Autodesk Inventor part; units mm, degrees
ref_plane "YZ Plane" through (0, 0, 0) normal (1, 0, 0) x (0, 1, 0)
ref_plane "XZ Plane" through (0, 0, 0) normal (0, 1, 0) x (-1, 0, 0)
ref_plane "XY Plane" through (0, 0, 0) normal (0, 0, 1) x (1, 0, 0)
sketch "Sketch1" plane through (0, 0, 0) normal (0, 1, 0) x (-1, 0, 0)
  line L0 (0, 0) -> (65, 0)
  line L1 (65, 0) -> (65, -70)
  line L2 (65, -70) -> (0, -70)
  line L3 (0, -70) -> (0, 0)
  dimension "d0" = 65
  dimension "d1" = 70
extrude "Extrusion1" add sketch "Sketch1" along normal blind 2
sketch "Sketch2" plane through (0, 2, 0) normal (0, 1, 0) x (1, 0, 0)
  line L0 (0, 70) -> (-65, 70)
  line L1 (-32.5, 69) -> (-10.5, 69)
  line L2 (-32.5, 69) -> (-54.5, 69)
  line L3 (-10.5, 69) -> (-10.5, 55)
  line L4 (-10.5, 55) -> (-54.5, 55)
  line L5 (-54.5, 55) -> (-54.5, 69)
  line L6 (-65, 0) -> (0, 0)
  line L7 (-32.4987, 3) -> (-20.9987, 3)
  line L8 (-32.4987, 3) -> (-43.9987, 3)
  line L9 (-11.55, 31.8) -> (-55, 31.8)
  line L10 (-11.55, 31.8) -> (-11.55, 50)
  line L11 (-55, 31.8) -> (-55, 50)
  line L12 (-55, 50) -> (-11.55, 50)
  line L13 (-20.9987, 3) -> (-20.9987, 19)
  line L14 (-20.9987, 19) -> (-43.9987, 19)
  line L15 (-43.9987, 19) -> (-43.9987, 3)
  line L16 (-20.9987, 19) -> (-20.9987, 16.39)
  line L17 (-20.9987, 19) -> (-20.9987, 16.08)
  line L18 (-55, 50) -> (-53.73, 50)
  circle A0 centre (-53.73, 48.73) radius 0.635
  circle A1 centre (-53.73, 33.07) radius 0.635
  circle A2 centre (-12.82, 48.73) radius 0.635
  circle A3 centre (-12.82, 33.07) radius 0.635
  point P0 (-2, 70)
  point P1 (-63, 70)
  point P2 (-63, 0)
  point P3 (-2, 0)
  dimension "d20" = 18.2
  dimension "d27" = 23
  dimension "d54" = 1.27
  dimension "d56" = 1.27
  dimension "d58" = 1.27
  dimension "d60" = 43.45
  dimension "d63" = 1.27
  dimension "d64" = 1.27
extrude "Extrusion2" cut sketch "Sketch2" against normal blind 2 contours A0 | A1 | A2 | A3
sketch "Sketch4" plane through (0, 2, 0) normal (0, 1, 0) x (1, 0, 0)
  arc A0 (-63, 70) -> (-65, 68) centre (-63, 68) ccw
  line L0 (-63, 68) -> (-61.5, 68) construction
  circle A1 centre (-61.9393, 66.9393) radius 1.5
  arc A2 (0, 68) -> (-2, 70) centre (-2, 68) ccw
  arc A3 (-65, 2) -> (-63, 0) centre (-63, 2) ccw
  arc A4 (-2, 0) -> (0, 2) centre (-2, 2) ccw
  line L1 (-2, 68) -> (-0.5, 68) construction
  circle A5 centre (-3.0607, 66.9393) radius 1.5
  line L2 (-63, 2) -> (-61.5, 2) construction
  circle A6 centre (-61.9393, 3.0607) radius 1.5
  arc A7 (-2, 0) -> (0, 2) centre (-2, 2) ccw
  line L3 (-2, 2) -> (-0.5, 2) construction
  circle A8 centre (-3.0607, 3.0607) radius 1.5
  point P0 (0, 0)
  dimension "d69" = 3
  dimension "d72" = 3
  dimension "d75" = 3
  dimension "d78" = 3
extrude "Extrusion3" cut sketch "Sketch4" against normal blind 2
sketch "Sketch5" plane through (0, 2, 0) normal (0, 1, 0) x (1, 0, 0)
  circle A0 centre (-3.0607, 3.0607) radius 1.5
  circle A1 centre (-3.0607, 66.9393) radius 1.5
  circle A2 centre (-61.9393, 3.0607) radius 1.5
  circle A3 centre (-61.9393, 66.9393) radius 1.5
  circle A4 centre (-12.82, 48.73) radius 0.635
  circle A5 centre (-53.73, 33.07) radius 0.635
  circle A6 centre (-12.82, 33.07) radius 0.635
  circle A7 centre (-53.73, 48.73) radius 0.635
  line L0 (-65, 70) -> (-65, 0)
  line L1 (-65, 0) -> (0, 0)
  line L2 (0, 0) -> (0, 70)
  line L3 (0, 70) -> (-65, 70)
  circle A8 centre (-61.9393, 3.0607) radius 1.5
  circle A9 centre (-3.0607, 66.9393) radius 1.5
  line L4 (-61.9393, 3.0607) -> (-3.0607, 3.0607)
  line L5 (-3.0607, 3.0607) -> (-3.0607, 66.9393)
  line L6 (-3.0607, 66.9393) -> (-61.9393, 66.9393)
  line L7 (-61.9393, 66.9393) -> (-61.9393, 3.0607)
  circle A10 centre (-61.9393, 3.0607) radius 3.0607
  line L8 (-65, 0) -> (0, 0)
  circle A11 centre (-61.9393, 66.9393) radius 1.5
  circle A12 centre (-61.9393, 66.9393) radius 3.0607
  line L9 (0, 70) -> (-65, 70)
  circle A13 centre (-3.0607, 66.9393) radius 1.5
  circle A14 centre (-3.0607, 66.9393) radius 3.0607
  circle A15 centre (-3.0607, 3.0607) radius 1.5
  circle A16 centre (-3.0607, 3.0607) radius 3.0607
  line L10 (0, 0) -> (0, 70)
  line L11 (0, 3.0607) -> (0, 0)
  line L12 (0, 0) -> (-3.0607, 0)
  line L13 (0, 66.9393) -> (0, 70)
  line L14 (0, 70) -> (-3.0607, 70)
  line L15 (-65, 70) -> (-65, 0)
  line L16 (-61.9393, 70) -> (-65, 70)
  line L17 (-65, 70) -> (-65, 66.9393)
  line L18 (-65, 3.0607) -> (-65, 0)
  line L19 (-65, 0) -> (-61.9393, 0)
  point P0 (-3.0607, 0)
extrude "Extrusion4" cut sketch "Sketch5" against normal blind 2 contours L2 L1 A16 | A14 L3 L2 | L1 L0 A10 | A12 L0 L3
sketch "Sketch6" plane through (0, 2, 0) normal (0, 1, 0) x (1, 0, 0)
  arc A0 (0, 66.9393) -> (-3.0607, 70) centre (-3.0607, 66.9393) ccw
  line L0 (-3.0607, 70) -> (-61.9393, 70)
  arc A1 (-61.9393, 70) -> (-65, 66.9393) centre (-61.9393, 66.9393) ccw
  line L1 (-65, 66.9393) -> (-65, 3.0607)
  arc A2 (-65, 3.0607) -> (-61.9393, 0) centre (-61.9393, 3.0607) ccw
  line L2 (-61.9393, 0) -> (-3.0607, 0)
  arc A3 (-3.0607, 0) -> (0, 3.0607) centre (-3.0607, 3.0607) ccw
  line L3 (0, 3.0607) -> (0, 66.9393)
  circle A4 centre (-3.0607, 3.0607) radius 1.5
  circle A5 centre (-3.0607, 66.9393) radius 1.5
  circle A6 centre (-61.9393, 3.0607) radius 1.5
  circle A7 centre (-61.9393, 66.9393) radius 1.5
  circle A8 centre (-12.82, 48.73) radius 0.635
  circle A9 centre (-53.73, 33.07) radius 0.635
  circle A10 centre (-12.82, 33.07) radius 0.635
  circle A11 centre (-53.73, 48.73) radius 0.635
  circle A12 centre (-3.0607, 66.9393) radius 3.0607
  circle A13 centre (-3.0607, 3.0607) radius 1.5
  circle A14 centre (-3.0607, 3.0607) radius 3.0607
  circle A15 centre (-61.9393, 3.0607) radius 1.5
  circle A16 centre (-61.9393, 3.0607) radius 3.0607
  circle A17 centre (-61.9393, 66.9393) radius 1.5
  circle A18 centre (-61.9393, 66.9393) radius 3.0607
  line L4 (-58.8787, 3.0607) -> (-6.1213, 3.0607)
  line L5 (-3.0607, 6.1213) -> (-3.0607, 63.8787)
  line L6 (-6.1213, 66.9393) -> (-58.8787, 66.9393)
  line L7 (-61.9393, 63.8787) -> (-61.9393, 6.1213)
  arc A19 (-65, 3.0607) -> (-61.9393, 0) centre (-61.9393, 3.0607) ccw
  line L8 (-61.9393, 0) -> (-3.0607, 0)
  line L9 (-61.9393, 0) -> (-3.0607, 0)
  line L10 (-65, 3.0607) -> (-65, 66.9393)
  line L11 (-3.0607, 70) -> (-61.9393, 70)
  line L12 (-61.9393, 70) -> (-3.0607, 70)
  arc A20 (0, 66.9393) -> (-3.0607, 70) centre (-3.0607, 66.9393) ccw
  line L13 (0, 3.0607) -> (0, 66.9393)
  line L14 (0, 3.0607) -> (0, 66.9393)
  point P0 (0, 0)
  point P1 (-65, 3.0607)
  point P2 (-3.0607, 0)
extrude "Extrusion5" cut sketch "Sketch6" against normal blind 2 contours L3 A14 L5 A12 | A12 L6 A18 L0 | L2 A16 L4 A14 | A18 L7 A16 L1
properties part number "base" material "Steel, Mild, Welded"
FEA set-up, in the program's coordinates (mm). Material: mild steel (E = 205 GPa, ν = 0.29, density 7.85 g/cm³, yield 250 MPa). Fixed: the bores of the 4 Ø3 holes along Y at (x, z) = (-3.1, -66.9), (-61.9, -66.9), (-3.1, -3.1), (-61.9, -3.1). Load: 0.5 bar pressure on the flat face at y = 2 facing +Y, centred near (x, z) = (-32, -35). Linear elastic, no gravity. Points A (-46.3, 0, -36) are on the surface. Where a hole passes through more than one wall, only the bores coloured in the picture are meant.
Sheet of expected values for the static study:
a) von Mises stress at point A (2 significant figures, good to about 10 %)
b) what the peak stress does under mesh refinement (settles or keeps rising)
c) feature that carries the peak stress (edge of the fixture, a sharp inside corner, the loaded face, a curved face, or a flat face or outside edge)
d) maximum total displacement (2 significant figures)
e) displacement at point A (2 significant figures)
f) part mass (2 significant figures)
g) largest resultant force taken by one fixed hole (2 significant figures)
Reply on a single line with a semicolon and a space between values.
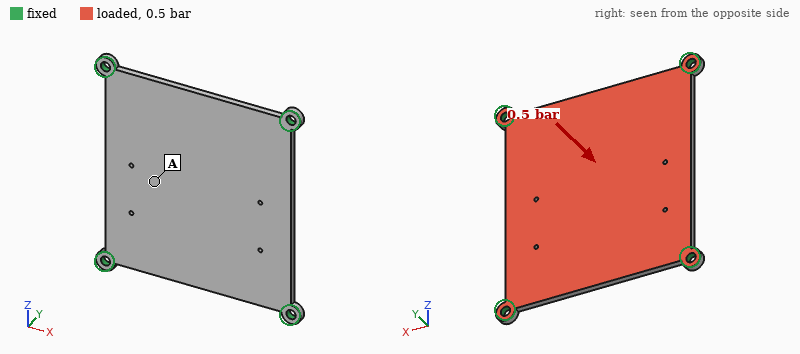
18 MPa; keeps rising; edge of the fixture; 48 µm; 44 µm; 60 g; 48 N
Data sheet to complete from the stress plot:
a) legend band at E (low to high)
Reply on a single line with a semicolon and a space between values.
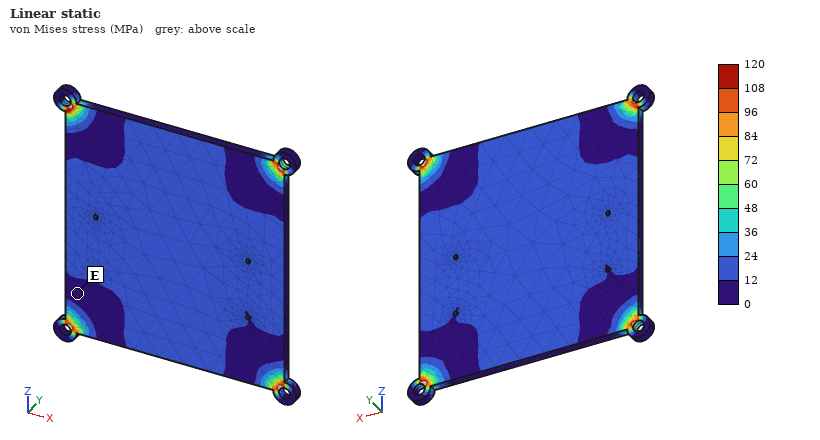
0 to 12 MPa
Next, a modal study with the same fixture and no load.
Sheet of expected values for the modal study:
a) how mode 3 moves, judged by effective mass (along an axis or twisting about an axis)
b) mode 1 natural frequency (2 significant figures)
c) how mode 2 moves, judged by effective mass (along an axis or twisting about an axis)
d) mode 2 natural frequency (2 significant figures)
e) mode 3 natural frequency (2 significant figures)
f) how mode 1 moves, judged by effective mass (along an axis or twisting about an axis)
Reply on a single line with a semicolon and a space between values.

twisting about X; 1500 Hz; twisting about Z; 2900 Hz; 3100 Hz; along Y
